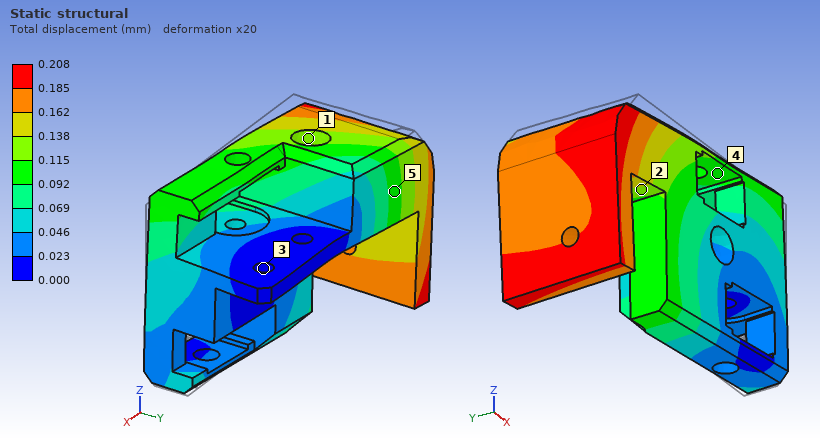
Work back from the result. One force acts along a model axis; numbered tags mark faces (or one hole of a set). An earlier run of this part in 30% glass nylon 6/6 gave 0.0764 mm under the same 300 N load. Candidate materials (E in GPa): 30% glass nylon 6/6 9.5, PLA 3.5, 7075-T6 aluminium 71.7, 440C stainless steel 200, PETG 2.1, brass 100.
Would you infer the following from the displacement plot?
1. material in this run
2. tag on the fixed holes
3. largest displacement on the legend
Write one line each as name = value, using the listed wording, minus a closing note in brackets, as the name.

material in this run = PLA
tag on the fixed holes = 3
largest displacement on the legend = 0.208 mm
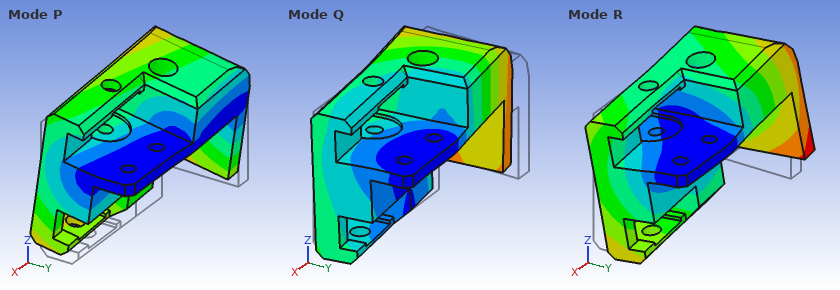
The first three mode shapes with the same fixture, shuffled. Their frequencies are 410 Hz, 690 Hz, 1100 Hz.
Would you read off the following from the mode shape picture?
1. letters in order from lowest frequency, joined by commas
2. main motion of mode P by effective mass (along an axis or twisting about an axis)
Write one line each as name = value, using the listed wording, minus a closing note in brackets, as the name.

letters in order from lowest frequency, joined by commas = P, R, Q
main motion of mode P by effective mass = along Z
